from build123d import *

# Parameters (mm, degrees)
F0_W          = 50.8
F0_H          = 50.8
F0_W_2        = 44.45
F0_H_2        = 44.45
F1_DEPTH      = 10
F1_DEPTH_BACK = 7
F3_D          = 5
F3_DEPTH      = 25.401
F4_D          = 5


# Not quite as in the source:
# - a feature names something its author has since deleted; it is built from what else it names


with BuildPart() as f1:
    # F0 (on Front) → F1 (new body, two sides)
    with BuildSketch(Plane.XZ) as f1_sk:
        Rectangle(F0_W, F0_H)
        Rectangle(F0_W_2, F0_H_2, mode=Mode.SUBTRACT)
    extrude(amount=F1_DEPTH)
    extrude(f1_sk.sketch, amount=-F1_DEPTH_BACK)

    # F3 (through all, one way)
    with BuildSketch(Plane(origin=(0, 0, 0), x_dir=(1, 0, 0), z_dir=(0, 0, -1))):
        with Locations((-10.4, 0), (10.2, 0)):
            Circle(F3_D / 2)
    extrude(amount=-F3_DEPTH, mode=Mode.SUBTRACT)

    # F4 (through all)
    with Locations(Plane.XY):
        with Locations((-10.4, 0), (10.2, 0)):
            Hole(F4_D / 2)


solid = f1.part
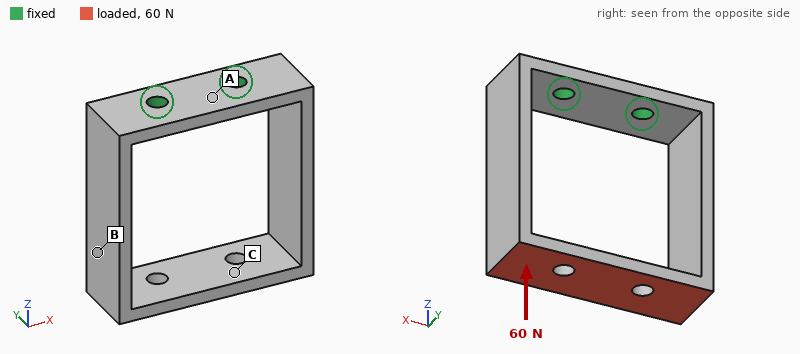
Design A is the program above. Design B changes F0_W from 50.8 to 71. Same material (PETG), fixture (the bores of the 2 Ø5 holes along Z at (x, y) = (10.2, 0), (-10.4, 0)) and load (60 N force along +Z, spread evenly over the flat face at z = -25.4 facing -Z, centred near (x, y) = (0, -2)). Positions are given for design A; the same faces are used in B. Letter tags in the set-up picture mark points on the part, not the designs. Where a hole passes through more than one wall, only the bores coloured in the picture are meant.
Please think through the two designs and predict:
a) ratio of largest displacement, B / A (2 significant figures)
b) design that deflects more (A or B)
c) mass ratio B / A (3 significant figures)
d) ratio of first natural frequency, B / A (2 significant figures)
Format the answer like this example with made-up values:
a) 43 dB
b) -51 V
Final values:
a) 0.36
b) A
c) 2.74
d) 0.74
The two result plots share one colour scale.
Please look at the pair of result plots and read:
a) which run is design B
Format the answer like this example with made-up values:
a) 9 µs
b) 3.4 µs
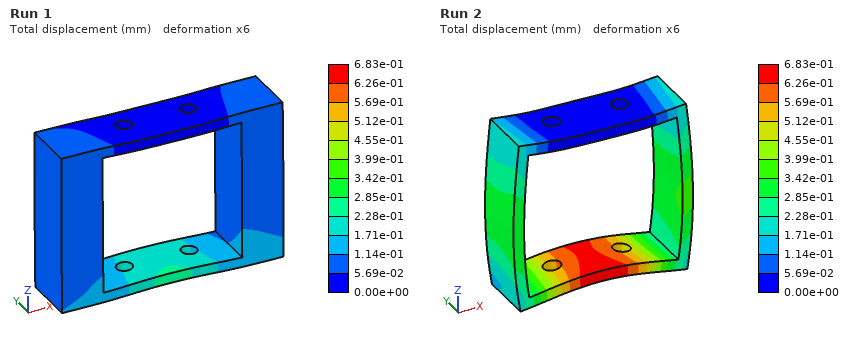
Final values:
a) Run 1
